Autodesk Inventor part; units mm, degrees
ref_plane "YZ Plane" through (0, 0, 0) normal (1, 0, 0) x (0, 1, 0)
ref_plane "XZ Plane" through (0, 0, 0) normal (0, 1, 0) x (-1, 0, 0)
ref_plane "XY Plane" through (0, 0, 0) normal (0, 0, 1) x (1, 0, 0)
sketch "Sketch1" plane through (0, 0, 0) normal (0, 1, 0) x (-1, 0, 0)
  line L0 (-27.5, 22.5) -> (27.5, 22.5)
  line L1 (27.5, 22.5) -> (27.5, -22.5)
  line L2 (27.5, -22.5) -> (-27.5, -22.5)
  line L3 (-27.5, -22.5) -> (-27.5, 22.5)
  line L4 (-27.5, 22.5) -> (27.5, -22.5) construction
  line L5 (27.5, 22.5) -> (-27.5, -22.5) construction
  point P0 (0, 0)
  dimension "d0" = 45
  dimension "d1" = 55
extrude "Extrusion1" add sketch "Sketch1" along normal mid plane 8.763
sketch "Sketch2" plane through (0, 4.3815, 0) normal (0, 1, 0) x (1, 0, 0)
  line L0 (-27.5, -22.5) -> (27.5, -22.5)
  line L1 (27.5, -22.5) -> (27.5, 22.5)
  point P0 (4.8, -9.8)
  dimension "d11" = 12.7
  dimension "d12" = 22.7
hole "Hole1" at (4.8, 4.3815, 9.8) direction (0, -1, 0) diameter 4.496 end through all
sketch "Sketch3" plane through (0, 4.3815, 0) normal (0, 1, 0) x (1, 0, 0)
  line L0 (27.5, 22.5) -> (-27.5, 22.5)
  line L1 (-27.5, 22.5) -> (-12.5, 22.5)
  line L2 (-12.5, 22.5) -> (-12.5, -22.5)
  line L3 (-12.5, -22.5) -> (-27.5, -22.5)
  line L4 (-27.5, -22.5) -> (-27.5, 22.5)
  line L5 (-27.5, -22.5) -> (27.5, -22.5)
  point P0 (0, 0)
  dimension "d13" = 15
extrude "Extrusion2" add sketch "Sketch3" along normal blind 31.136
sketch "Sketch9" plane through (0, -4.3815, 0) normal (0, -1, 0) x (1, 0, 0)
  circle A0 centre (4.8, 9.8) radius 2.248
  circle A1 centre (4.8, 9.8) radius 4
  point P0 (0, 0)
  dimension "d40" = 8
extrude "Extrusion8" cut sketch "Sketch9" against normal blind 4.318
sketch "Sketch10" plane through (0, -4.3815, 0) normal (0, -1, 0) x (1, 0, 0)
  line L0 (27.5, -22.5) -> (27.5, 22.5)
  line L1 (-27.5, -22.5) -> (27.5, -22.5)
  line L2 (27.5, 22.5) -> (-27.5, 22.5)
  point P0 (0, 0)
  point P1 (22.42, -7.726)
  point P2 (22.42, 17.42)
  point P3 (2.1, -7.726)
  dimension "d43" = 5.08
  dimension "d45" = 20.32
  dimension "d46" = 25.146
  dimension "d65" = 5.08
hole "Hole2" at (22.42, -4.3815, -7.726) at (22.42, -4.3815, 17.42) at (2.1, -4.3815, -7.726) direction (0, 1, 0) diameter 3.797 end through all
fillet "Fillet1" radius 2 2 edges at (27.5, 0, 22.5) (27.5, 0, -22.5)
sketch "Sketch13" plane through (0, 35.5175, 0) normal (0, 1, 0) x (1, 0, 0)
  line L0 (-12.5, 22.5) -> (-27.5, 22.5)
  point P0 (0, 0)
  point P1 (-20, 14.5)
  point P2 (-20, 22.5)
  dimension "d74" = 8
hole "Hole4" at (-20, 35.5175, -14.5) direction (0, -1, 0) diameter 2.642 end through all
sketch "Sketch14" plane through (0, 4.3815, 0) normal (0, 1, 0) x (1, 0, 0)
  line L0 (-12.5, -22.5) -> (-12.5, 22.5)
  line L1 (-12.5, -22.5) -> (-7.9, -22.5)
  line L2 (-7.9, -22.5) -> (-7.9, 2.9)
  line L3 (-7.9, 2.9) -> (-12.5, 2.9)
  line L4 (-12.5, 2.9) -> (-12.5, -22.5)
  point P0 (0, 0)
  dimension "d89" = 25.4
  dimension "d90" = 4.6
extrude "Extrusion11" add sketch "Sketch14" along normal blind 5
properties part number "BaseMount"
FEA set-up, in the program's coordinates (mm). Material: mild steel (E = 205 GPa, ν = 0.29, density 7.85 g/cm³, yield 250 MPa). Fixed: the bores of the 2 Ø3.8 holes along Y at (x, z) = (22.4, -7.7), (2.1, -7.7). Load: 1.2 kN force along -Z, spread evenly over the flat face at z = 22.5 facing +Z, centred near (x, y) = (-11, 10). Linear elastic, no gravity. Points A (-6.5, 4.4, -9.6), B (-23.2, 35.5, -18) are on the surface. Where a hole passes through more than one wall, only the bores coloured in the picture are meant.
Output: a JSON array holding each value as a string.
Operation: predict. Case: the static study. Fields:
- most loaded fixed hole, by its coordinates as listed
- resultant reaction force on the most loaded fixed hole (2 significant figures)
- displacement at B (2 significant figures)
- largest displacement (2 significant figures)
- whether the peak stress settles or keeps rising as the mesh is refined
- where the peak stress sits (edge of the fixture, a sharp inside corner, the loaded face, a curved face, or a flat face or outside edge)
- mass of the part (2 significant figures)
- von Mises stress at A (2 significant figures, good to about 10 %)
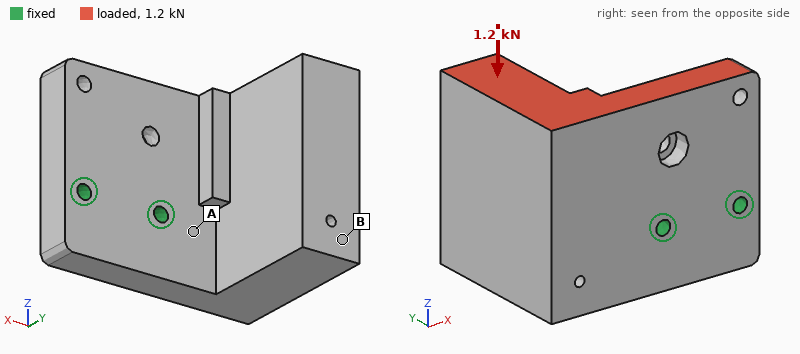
["(2.1, -7.7)", "1.8 kN", "16 µm", "19 µm", "keeps rising", "edge of the fixture", "330 g", "20 MPa"]
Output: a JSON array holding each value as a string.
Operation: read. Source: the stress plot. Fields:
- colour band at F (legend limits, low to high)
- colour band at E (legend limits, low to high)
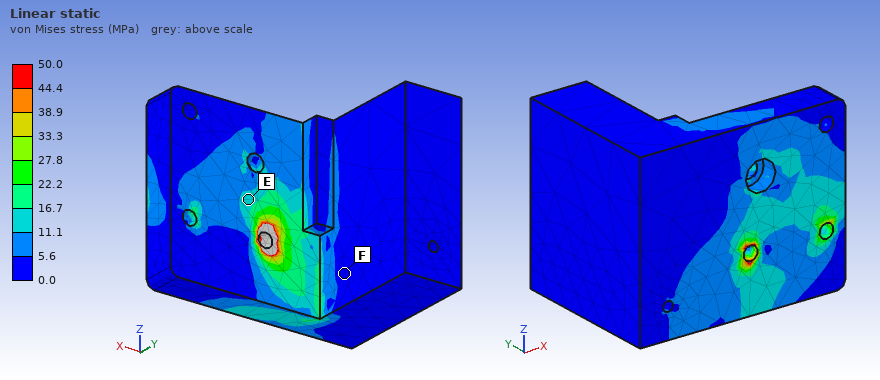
["0.0 to 5.6 MPa", "11.1 to 16.7 MPa"]
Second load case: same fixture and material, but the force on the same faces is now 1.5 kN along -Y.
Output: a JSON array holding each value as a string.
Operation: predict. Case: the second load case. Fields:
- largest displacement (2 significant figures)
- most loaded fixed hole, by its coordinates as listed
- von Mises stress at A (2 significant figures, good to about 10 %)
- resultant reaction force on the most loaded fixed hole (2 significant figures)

["75 µm", "(2.1, -7.7)", "56 MPa", "1.8 kN"]
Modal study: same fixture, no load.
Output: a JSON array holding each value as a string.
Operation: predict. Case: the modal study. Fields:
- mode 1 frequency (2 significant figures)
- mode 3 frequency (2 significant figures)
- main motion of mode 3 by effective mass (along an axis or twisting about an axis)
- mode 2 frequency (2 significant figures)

["1900 Hz", "6400 Hz", "along Z", "2700 Hz"]
